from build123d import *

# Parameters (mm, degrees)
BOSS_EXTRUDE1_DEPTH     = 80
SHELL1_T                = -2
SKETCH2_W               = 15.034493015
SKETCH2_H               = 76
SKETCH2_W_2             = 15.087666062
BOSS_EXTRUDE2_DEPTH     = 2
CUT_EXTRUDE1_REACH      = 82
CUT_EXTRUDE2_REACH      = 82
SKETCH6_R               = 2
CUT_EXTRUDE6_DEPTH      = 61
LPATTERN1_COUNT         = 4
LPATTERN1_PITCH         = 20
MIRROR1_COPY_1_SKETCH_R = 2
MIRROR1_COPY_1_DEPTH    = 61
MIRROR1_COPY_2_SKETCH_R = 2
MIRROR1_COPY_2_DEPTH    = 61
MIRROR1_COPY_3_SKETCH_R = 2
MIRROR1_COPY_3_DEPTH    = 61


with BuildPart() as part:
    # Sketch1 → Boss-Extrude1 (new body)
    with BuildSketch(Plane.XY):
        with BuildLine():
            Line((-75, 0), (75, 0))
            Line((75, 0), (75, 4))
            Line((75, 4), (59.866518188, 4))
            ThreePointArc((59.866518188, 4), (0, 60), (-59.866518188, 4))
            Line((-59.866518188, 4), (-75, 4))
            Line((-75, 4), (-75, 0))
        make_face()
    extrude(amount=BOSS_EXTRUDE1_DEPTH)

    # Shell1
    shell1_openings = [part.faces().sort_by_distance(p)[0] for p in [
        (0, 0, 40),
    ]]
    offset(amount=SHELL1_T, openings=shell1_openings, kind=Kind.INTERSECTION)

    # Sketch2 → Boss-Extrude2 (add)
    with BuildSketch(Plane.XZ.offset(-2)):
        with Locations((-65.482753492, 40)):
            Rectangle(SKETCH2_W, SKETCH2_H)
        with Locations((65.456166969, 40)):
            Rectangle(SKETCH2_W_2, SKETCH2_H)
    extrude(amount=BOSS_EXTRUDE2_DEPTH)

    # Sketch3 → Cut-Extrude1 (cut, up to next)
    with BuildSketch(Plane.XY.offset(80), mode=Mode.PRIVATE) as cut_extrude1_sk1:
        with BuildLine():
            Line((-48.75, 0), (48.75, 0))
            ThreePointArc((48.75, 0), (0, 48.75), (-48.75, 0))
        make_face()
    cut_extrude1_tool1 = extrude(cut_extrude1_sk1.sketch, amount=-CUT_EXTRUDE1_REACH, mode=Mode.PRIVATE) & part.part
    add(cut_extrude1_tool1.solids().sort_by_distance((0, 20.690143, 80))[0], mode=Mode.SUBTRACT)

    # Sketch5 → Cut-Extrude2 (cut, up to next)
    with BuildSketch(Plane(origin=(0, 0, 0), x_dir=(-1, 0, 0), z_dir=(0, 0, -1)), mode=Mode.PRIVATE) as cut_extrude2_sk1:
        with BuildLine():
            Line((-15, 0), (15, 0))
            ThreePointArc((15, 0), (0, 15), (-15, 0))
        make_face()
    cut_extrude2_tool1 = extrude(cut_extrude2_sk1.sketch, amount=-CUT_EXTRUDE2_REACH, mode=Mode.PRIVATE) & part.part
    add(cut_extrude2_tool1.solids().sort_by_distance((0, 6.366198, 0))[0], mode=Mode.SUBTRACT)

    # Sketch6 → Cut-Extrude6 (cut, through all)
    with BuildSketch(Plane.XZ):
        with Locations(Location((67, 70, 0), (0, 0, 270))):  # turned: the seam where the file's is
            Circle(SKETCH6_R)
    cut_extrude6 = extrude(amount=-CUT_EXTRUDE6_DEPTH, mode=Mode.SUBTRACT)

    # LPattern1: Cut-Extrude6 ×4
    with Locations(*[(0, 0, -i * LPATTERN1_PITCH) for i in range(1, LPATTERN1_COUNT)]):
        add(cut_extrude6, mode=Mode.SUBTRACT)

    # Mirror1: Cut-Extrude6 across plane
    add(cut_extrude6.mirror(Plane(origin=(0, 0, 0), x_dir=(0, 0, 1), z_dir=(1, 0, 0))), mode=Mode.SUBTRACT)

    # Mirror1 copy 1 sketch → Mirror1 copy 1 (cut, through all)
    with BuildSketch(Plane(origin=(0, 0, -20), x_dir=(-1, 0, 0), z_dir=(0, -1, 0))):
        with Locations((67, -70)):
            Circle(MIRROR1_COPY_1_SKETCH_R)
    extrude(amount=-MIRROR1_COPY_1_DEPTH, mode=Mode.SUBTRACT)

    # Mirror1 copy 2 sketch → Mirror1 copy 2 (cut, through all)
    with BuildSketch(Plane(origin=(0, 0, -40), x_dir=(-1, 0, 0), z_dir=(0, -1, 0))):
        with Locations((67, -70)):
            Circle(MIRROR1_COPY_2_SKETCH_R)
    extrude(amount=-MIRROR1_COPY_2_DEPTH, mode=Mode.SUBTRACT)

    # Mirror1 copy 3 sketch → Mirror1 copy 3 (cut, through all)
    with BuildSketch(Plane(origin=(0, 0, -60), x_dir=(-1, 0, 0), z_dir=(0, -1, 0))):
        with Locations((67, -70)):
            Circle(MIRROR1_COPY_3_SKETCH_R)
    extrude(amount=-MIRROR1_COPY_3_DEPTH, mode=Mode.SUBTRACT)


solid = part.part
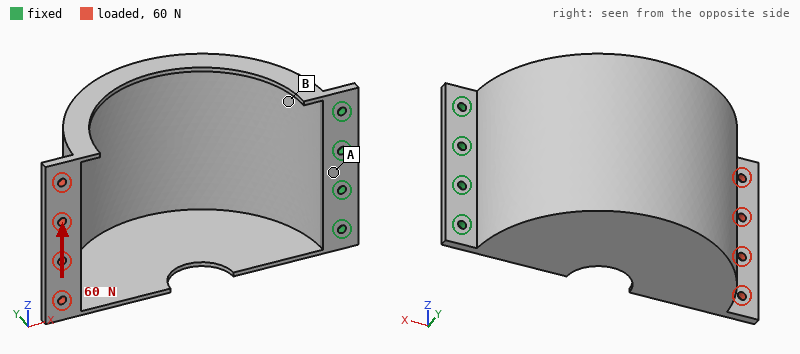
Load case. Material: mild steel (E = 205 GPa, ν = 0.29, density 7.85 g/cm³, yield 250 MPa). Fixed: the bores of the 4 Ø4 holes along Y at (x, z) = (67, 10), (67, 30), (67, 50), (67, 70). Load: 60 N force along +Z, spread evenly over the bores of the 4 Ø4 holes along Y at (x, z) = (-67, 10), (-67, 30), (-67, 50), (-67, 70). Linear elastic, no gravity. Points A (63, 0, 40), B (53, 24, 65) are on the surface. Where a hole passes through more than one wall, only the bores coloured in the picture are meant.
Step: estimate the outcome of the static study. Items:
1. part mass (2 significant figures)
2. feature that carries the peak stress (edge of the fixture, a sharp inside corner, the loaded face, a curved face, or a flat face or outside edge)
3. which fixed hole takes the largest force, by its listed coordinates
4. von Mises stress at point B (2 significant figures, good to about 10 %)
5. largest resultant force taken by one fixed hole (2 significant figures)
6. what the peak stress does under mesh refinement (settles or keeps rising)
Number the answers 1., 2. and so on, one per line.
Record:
1. 410 g
2. a sharp inside corner
3. (67, 10)
4. 20 MPa
5. 160 N
6. keeps rising
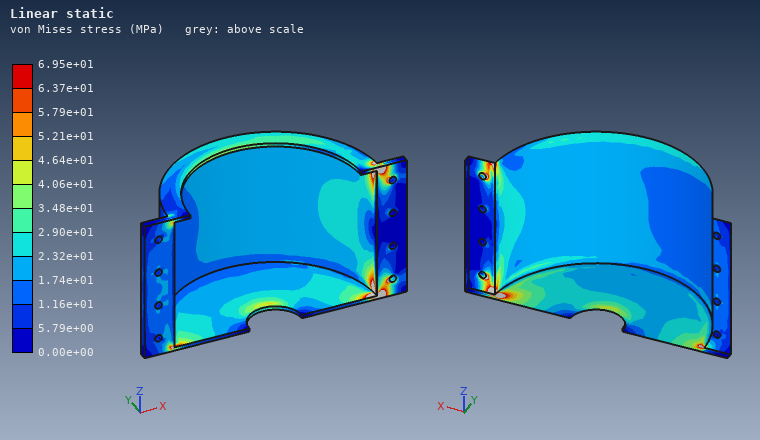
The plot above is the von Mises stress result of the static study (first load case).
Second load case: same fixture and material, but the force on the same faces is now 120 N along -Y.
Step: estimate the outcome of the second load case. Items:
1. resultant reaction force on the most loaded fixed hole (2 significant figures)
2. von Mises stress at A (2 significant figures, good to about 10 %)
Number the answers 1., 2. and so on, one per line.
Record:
1. 370 N
2. 28 MPa
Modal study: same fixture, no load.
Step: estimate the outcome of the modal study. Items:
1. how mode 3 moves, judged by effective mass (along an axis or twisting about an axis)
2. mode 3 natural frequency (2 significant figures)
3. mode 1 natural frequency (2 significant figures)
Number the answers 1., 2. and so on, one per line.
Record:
1. along X
2. 530 Hz
3. 130 Hz
